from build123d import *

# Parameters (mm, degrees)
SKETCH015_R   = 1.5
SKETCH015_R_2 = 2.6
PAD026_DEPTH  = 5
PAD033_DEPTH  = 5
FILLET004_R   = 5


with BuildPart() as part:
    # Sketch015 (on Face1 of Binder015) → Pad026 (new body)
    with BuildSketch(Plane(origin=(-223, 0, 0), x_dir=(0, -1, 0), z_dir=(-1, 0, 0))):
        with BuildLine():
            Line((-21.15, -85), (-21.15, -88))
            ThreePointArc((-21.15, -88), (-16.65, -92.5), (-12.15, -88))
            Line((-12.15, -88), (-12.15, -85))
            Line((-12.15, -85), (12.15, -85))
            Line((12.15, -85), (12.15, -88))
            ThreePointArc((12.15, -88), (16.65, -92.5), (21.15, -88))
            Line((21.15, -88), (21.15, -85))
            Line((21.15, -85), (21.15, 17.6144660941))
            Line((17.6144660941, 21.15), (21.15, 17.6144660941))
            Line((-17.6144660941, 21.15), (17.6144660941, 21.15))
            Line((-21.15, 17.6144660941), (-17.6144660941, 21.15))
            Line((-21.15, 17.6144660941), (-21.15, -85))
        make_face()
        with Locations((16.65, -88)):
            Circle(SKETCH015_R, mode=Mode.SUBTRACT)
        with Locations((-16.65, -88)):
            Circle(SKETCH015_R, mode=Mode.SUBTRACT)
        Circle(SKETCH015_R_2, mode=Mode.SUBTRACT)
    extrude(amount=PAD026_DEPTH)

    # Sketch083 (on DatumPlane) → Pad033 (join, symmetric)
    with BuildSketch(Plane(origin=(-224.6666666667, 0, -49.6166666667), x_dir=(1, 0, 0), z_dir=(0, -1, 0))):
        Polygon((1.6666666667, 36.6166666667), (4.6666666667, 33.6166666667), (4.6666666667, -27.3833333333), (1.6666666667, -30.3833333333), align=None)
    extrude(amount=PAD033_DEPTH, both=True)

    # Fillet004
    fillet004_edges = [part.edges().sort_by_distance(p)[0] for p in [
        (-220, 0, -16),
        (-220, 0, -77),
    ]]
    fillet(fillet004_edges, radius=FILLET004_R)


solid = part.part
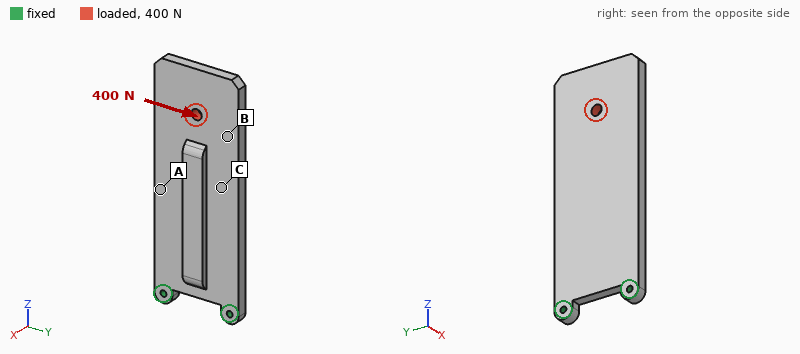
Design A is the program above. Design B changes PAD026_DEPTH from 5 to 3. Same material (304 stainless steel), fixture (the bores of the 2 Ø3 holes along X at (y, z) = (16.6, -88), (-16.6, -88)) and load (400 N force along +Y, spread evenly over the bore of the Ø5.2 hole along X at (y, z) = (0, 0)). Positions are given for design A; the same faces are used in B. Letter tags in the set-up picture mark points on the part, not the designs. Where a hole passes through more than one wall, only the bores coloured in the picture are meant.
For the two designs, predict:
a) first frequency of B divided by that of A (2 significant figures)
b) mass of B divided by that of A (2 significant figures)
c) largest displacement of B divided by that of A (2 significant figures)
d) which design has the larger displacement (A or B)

0.65
0.63
1.7
B
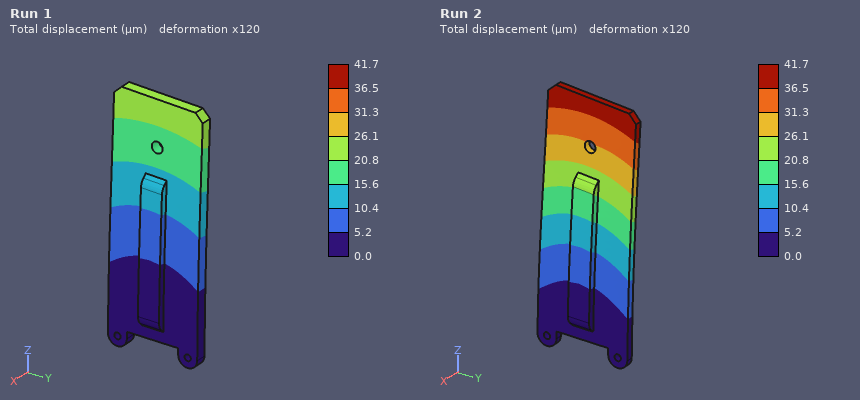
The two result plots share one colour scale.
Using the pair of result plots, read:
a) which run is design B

Run 2
